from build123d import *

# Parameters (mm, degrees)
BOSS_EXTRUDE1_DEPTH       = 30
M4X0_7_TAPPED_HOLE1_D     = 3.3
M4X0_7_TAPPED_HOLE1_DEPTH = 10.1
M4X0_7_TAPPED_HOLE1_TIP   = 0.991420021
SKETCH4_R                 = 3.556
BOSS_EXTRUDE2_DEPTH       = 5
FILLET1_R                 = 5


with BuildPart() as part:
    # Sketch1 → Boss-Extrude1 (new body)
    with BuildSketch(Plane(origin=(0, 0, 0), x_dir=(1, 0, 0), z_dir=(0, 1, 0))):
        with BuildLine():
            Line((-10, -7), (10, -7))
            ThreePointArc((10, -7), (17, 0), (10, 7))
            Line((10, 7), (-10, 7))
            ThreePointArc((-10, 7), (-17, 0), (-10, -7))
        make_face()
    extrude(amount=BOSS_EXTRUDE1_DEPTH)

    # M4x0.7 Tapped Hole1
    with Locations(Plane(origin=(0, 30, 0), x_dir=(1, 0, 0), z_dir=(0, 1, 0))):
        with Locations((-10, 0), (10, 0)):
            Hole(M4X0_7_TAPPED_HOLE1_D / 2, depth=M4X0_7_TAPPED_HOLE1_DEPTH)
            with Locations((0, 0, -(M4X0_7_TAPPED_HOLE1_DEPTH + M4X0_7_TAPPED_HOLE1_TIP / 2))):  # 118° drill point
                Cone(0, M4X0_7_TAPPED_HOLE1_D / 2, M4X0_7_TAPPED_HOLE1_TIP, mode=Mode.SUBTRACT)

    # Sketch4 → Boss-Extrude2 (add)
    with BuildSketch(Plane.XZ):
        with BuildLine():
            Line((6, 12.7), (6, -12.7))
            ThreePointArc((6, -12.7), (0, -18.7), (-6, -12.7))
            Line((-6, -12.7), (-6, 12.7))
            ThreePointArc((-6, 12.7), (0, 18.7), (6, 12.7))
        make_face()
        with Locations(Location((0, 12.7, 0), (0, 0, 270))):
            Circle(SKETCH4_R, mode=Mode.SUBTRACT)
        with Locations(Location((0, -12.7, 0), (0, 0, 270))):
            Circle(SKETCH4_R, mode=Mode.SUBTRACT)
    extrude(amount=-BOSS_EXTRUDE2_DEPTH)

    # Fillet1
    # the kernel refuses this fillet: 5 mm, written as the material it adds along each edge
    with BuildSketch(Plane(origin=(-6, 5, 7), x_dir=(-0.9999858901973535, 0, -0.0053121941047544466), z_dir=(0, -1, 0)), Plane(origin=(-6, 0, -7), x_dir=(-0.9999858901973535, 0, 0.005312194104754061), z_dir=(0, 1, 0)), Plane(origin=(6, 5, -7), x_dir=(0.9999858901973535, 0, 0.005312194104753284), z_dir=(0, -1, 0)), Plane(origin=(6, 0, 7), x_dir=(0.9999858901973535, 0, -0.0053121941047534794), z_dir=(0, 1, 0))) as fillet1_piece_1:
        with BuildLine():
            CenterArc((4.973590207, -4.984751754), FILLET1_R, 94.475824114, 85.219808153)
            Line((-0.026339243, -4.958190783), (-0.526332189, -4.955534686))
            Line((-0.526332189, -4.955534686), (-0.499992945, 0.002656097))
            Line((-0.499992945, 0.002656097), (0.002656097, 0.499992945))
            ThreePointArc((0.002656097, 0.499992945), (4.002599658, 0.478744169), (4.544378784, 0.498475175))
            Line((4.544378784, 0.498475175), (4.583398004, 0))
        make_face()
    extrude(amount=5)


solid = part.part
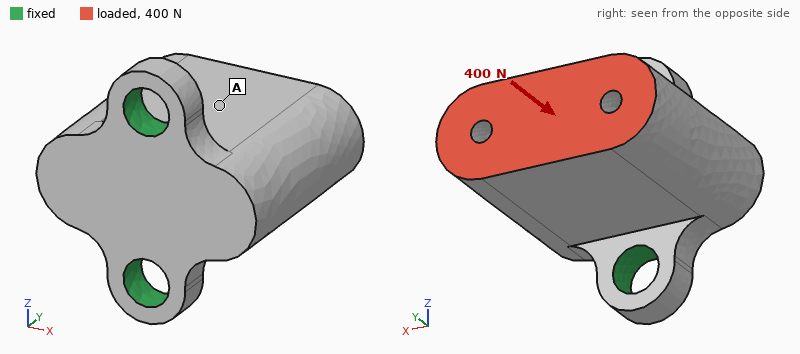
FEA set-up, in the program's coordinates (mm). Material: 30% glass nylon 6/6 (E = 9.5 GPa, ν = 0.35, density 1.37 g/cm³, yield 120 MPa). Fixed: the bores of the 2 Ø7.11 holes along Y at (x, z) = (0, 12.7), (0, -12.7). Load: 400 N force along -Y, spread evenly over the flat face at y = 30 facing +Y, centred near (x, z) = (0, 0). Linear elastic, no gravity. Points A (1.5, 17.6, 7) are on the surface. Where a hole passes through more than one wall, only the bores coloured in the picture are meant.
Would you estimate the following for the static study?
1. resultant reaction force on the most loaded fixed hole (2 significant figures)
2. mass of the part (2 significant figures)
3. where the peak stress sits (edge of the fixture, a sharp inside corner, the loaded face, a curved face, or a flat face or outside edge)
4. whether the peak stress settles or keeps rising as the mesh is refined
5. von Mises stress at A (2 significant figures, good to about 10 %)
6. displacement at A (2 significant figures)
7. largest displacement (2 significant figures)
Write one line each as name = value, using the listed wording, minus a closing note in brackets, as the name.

resultant reaction force on the most loaded fixed hole = 210 N
mass of the part = 19 g
where the peak stress sits = edge of the fixture
whether the peak stress settles or keeps rising as the mesh is refined = keeps rising
von Mises stress at A = 1.3 MPa
displacement at A = 8.1 µm
largest displacement = 9.7 µm
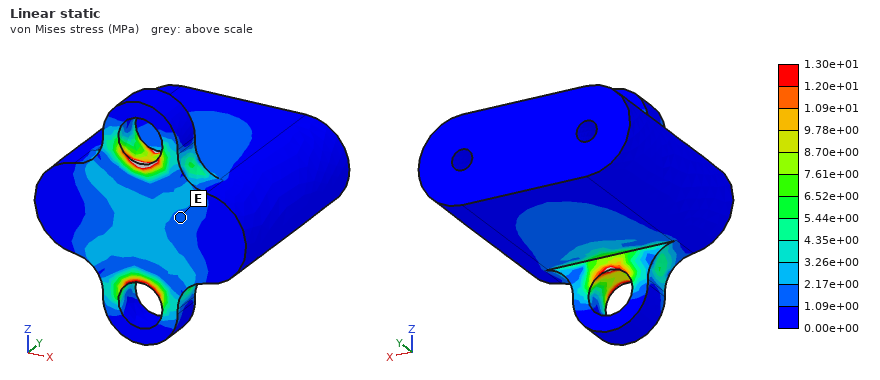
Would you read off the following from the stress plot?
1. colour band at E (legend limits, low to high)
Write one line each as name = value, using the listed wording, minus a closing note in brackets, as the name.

colour band at E = 1.09e+00 to 2.17e+00 MPa
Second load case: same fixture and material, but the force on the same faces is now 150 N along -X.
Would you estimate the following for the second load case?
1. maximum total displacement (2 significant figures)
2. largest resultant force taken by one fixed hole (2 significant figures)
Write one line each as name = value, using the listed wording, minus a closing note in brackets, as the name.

maximum total displacement = 0.14 mm
largest resultant force taken by one fixed hole = 75 N
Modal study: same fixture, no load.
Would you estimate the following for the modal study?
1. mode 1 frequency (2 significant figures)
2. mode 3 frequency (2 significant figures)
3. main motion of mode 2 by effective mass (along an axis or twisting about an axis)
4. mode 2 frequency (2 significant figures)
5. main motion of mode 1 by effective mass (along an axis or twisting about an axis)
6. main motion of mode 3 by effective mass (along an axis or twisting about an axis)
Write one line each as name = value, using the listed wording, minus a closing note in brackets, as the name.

mode 1 frequency = 2100 Hz
mode 3 frequency = 8600 Hz
main motion of mode 2 by effective mass = along Z
mode 2 frequency = 4300 Hz
main motion of mode 1 by effective mass = along X
main motion of mode 3 by effective mass = along Y
